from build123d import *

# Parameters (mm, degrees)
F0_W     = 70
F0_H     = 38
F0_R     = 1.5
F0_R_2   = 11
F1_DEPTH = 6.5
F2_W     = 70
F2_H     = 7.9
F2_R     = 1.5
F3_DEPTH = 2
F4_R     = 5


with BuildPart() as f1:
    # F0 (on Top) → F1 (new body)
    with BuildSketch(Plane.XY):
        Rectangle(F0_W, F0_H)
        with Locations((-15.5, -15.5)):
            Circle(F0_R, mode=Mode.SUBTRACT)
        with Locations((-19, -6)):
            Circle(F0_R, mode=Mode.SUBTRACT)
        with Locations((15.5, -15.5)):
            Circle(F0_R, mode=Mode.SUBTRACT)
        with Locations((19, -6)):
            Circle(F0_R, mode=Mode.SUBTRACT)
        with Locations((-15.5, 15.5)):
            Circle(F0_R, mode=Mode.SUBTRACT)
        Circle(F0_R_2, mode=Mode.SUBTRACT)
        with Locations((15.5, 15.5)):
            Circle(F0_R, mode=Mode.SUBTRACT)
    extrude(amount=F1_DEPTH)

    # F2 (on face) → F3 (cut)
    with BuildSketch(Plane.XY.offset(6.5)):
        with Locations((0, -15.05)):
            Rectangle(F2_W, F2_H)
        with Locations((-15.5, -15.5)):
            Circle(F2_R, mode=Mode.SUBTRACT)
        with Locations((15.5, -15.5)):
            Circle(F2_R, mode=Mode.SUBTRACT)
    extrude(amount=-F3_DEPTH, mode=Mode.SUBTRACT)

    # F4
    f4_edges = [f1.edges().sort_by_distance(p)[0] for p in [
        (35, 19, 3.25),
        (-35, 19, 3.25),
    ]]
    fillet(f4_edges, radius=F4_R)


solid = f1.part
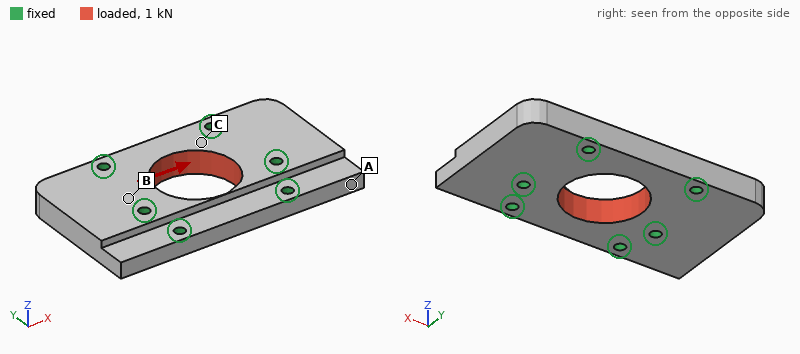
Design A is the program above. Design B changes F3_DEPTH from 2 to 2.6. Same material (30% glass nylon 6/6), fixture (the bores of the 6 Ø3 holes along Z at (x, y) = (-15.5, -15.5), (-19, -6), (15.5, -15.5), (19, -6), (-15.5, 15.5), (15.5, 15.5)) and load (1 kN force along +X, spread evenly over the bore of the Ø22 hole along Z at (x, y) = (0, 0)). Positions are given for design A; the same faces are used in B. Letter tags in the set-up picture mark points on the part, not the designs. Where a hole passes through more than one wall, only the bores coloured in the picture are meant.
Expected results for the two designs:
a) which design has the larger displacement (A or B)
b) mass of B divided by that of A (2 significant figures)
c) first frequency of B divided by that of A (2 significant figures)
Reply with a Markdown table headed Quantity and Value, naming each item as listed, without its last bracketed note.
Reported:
| Quantity | Value |
|---|---|
| which design has the larger displacement | B |
| mass of B divided by that of A | 0.98 |
| first frequency of B divided by that of A | 1.00 |
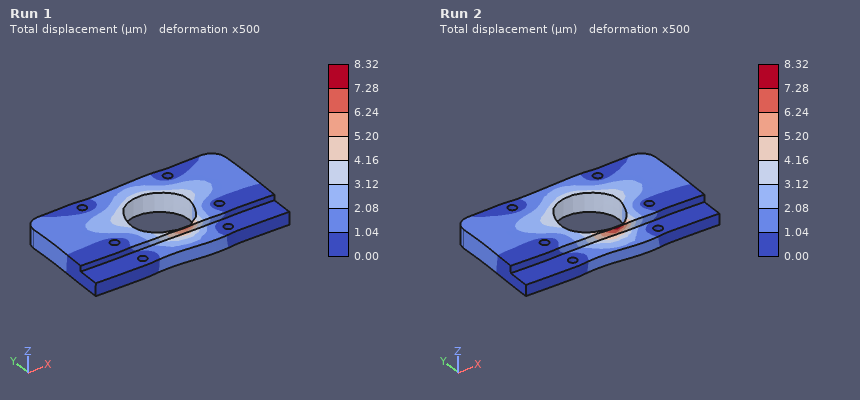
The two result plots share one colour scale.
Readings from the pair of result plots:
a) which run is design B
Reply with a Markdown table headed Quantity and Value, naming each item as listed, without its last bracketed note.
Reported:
| Quantity | Value |
|---|---|
| which run is design B | Run 2 |
